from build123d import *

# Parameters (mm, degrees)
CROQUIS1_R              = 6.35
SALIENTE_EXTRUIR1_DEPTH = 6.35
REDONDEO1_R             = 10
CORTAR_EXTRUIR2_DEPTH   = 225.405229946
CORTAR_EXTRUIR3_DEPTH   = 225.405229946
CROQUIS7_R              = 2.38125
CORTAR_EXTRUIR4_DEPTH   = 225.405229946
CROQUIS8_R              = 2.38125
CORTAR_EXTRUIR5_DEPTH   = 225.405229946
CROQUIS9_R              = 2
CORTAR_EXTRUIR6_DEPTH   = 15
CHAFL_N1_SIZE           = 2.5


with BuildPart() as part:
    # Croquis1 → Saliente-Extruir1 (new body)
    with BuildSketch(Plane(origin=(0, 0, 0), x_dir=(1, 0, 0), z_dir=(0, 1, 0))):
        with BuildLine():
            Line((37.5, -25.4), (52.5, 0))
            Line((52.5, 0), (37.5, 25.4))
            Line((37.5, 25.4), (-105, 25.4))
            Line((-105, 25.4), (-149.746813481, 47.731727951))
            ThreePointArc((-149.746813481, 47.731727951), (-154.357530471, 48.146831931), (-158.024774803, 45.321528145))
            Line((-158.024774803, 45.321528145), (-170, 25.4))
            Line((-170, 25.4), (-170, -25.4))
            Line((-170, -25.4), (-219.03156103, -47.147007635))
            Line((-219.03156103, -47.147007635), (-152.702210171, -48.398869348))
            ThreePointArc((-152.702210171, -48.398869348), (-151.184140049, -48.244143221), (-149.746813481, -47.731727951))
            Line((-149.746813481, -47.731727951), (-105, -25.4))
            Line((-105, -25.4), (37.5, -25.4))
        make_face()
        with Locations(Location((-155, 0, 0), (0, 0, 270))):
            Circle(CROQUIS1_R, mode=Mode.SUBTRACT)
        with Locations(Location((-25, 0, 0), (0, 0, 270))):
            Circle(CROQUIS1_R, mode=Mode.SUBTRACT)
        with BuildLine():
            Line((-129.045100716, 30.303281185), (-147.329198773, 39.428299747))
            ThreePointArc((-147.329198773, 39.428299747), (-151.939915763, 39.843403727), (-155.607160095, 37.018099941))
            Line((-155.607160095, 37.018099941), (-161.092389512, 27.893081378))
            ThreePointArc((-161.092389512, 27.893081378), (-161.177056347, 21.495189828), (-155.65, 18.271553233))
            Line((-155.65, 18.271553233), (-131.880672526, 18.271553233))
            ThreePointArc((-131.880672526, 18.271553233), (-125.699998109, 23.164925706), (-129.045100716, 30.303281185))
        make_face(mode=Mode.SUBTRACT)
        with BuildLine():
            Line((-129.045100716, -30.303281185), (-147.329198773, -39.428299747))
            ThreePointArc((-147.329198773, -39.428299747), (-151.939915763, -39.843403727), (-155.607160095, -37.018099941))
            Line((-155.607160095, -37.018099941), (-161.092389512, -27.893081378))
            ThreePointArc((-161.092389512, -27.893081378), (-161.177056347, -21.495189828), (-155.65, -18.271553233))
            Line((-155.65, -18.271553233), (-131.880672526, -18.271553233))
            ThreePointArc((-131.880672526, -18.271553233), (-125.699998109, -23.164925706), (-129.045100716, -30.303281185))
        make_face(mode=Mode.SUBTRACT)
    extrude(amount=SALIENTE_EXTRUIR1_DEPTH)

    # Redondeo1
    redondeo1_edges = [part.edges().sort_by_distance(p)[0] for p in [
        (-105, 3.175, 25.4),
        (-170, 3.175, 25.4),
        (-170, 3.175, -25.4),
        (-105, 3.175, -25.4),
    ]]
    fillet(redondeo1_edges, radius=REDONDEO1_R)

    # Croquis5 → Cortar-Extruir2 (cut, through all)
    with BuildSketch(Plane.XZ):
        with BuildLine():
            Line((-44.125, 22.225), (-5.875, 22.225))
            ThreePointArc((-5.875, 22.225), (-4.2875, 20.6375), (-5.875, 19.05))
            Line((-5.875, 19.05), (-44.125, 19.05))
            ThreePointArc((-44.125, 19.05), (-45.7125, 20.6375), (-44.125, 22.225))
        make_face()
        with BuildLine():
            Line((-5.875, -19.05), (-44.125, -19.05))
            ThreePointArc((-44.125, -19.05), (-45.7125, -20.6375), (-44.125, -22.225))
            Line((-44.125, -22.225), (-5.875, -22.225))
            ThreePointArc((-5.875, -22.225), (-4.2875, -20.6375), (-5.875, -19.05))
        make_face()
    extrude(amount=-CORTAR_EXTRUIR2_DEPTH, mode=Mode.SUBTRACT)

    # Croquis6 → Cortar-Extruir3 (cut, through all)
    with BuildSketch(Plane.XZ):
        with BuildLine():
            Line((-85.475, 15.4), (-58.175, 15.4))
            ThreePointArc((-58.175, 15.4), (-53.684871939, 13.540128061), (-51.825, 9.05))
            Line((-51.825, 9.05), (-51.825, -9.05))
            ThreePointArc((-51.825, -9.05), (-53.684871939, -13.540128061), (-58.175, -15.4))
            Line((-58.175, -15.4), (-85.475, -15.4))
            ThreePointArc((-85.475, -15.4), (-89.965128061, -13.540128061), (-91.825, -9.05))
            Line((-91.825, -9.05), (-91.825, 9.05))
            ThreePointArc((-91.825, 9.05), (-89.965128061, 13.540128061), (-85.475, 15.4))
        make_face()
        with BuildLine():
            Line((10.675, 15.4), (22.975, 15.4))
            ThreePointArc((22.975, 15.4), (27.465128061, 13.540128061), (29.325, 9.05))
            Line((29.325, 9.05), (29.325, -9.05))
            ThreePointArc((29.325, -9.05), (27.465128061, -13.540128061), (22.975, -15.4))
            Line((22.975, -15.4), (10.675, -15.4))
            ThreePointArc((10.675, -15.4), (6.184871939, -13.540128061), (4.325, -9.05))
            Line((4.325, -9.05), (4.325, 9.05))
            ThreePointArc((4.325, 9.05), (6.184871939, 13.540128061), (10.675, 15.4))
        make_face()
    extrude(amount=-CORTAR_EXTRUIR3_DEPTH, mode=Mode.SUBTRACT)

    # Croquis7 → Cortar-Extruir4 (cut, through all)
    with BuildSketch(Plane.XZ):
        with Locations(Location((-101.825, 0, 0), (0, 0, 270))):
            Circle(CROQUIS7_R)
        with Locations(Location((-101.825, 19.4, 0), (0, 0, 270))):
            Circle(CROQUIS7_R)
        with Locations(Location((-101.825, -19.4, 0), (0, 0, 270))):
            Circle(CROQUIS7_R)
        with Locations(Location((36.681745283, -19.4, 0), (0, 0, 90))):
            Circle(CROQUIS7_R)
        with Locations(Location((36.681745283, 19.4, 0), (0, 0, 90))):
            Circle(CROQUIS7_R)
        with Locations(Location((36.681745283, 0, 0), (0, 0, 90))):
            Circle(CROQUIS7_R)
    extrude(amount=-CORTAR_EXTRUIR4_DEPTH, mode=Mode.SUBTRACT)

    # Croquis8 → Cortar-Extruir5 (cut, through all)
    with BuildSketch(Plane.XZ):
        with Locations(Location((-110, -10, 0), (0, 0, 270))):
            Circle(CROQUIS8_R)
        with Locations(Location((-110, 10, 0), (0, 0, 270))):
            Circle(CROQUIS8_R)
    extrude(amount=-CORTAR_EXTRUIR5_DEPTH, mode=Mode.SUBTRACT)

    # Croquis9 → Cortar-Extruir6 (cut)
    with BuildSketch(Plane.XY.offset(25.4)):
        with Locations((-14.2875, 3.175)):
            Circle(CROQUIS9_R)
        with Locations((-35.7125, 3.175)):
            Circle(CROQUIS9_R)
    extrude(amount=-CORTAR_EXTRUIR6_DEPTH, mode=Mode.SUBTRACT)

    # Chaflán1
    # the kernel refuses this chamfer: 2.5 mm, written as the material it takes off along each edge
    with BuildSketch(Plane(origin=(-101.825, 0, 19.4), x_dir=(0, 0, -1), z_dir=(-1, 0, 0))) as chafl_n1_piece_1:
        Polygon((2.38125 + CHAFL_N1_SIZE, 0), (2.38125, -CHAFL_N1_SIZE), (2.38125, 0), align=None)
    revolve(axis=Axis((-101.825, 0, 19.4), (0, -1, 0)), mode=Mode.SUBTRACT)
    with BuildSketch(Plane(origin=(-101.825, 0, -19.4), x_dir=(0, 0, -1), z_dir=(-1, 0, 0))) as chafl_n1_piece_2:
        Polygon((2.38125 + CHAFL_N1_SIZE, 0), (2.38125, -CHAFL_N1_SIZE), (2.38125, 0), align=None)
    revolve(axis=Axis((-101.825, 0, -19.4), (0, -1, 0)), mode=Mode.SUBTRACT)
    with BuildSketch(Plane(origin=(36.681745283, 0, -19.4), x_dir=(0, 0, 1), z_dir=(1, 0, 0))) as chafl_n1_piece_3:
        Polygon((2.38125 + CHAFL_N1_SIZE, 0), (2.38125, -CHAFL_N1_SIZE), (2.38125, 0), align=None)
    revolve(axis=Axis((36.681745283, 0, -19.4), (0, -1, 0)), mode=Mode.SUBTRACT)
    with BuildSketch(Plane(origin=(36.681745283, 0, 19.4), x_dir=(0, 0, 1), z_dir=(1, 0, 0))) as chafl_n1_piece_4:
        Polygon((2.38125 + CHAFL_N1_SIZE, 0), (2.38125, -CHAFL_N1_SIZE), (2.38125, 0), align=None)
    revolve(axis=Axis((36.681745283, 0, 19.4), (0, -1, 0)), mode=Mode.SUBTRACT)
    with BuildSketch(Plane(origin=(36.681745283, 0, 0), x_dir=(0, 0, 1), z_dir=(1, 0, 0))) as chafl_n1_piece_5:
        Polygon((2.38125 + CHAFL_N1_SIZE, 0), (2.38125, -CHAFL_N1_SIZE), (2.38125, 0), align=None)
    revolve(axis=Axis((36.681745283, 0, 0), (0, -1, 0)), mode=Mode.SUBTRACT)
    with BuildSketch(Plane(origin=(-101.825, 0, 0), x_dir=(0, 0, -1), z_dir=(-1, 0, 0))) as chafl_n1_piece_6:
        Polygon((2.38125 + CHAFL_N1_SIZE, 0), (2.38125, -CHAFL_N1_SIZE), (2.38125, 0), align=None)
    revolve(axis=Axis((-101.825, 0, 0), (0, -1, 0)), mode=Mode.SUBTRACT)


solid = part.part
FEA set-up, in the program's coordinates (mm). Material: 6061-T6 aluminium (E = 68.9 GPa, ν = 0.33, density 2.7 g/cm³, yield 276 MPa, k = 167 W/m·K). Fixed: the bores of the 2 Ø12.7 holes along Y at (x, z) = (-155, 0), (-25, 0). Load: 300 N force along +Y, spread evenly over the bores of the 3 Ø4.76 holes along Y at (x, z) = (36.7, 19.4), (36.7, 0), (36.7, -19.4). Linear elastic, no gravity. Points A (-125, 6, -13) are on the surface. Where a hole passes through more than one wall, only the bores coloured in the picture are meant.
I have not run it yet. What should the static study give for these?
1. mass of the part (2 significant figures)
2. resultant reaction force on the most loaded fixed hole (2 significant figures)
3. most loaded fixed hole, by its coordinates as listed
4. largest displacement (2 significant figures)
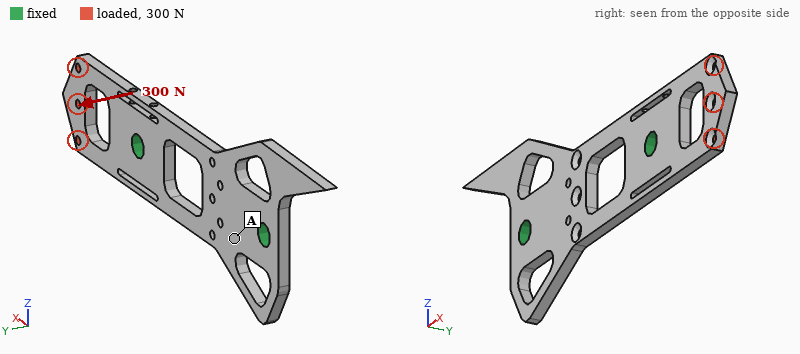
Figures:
160 g
300 N
(-25, 0)
0.59 mm
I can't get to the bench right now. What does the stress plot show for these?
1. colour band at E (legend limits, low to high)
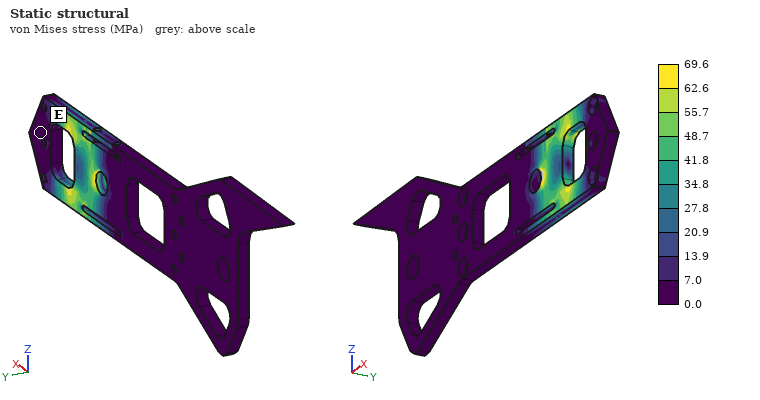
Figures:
0.0 to 7.0 MPa
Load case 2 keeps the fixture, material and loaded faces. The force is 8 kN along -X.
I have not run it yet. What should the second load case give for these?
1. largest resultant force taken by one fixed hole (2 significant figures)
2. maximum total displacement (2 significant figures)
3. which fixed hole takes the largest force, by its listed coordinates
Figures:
7.3 kN
0.63 mm
(-25, 0)
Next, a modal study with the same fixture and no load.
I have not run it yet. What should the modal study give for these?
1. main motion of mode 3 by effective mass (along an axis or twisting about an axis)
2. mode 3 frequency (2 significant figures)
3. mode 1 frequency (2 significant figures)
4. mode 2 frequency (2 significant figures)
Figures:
along Y
2000 Hz
1100 Hz
1300 Hz
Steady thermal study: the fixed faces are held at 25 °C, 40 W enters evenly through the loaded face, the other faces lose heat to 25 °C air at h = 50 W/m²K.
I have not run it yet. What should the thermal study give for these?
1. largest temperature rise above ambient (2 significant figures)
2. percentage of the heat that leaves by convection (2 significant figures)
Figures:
71 K
34 %
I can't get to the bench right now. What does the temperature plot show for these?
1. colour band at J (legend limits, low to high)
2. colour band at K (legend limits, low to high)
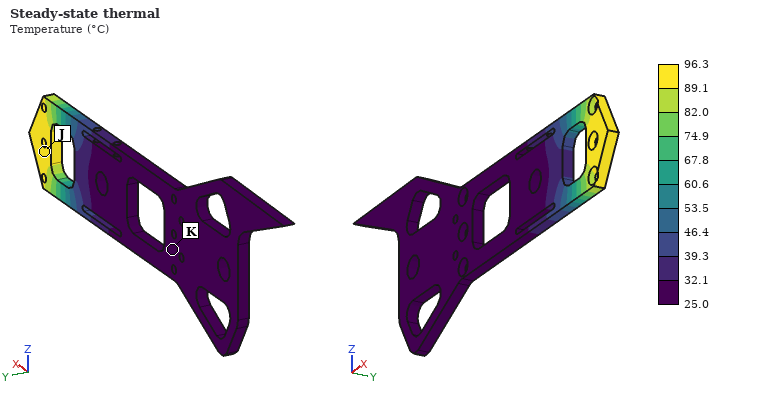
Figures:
89.1 to 96.3 °C
25.0 to 32.1 °C
